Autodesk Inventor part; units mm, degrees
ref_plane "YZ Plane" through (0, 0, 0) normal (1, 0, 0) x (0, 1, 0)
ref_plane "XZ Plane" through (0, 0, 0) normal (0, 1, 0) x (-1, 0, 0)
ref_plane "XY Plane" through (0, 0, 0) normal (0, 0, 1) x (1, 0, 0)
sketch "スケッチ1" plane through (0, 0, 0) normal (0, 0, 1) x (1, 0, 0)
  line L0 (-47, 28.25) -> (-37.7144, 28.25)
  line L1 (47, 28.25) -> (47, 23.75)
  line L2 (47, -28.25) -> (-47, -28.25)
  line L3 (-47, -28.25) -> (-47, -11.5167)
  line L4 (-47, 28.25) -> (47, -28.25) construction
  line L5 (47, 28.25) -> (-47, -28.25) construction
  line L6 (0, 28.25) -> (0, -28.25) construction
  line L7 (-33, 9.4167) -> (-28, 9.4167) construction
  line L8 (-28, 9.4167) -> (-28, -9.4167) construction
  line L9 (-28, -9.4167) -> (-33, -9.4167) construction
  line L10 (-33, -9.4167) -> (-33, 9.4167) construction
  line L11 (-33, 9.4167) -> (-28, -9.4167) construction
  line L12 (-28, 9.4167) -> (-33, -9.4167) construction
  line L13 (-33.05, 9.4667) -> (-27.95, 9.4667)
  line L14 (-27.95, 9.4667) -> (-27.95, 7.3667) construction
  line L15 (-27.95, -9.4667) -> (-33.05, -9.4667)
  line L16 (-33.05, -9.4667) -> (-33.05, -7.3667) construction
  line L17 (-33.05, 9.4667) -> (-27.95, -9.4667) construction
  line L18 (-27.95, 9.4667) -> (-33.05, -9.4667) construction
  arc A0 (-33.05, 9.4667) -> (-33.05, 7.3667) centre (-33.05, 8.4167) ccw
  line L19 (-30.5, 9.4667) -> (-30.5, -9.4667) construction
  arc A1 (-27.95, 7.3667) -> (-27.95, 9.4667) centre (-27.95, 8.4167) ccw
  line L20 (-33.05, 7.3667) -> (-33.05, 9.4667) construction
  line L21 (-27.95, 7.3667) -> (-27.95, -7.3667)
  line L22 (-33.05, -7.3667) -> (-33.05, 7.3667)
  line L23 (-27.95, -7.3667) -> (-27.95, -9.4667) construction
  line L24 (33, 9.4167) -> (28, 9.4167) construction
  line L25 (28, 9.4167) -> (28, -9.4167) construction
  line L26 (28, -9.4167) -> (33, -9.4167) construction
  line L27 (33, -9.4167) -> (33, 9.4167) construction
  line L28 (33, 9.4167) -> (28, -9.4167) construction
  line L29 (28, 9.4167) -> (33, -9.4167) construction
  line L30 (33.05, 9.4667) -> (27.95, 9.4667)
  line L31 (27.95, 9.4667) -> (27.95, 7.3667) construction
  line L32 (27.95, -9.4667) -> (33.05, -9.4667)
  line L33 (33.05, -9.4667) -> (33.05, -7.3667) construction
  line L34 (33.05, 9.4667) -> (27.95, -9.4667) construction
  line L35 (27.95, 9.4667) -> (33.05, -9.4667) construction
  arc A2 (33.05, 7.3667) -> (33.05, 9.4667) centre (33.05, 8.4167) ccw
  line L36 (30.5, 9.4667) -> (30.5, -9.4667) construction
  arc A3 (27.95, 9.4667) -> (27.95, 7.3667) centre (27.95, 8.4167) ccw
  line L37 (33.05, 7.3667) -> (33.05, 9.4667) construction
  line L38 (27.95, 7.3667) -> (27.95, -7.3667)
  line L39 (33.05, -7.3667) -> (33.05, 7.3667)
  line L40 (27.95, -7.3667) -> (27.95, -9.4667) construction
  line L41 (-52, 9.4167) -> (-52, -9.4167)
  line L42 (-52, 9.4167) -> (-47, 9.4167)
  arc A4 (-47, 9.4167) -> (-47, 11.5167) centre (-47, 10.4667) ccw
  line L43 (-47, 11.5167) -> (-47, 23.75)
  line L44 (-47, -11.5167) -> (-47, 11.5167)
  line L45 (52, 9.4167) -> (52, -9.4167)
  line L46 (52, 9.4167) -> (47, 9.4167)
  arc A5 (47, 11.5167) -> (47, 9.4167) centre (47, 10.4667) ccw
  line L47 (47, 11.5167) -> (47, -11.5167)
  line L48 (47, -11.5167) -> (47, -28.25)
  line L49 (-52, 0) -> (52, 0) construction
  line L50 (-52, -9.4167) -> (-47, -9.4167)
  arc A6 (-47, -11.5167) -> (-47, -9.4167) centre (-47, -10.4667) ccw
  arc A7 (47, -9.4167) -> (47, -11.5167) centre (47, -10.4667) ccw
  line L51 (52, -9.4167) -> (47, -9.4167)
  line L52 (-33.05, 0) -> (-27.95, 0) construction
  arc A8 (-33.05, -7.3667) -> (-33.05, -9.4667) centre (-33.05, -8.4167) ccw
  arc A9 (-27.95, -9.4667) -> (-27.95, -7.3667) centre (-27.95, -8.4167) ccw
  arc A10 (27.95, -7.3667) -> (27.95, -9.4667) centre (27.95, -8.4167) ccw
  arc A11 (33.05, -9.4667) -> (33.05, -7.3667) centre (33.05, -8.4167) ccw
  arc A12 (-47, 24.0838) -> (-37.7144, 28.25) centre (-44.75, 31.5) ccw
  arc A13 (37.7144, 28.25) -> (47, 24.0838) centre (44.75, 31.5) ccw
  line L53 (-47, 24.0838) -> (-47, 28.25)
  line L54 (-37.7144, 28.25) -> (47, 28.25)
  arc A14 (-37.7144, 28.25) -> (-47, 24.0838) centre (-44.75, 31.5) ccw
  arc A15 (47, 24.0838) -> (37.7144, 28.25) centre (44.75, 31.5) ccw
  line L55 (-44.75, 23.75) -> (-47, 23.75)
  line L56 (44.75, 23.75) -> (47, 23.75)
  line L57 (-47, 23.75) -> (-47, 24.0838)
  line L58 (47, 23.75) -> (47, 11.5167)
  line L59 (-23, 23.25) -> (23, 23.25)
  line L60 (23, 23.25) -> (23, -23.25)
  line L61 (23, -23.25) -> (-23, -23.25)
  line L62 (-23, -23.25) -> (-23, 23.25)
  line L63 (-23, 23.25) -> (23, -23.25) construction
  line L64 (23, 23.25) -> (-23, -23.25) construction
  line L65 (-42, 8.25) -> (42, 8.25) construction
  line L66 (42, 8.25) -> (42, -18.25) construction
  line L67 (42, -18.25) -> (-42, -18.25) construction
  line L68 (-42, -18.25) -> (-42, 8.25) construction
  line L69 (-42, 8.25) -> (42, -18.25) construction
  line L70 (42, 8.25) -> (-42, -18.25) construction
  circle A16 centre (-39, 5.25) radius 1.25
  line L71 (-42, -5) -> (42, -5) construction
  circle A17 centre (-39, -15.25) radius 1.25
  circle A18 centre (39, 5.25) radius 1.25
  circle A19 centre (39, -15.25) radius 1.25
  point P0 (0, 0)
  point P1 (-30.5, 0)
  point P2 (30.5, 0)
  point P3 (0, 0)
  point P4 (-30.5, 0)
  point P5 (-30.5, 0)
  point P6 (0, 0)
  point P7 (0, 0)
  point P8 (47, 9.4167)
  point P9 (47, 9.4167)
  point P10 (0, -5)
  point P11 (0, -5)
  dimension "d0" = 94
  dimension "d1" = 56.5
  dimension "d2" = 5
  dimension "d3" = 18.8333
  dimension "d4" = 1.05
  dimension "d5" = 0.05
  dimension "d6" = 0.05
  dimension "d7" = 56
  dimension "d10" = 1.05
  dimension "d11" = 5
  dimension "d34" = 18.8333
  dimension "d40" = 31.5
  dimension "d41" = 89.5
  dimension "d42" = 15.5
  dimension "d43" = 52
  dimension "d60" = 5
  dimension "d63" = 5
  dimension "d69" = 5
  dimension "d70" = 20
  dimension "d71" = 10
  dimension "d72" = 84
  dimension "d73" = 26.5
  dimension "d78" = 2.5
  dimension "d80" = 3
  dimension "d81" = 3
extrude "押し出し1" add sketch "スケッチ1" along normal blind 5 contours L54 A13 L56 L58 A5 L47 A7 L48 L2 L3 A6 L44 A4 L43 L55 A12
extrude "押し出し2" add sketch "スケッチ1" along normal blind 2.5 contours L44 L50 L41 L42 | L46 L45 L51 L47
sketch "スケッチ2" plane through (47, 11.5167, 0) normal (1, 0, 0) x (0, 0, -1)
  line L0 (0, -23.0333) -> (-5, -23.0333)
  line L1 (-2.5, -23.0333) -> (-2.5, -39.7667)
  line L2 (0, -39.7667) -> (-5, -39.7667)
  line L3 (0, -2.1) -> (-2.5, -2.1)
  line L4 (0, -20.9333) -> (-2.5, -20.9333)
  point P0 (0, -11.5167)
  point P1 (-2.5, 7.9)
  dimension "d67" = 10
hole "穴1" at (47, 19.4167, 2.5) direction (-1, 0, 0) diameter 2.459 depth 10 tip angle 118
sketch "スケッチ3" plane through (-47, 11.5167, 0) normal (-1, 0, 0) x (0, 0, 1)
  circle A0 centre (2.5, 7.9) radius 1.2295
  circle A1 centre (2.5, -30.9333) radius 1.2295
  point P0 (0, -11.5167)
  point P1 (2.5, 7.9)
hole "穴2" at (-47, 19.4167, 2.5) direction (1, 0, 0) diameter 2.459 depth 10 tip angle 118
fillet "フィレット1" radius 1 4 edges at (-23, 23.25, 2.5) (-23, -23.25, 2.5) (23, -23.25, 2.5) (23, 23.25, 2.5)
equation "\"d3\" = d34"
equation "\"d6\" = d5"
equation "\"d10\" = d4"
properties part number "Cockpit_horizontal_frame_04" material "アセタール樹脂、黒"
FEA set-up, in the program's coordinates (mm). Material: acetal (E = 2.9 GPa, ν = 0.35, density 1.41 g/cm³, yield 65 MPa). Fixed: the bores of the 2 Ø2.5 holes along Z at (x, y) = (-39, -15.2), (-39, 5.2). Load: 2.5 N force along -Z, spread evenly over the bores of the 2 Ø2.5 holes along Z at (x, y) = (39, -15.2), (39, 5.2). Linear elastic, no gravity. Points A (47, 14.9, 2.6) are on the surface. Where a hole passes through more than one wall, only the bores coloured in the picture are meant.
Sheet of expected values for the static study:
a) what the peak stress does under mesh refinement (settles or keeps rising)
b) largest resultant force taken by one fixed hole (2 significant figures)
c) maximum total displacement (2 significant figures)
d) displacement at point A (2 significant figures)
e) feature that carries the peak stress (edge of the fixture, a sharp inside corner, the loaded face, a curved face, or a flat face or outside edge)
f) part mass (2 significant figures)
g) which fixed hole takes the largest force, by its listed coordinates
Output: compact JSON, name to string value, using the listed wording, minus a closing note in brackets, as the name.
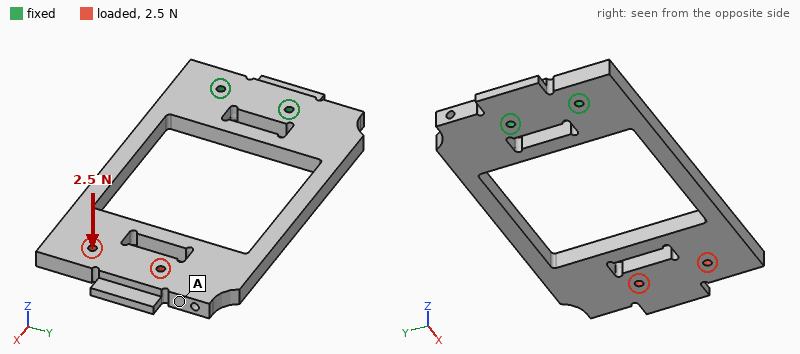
{"what the peak stress does under mesh refinement": "keeps rising", "largest resultant force taken by one fixed hole": "2.2 N", "maximum total displacement": "1.3 mm", "displacement at point A": "1.2 mm", "feature that carries the peak stress": "a sharp inside corner", "part mass": "21 g", "which fixed hole takes the largest force, by its listed coordinates": "(-39, -15.2)"}
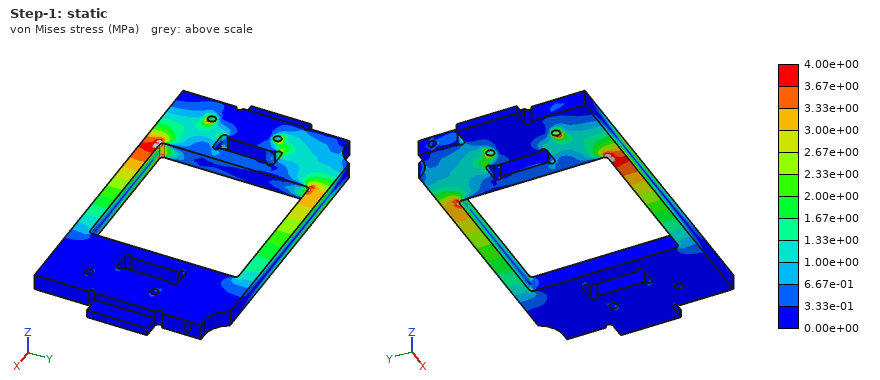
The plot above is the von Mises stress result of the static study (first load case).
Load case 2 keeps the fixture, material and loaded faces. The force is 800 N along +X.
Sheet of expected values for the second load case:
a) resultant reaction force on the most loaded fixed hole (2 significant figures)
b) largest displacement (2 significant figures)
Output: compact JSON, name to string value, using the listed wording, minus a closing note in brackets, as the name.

{"resultant reaction force on the most loaded fixed hole": "430 N", "largest displacement": "0.69 mm"}
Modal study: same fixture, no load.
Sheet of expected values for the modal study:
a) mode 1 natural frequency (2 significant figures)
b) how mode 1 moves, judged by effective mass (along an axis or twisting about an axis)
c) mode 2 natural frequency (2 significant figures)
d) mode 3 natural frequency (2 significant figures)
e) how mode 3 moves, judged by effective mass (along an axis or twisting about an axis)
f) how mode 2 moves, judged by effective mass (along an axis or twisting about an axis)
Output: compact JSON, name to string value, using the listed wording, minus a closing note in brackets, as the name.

{"mode 1 natural frequency": "86 Hz", "how mode 1 moves, judged by effective mass": "along Z", "mode 2 natural frequency": "240 Hz", "mode 3 natural frequency": "290 Hz", "how mode 3 moves, judged by effective mass": "twisting about X", "how mode 2 moves, judged by effective mass": "along Y"}
